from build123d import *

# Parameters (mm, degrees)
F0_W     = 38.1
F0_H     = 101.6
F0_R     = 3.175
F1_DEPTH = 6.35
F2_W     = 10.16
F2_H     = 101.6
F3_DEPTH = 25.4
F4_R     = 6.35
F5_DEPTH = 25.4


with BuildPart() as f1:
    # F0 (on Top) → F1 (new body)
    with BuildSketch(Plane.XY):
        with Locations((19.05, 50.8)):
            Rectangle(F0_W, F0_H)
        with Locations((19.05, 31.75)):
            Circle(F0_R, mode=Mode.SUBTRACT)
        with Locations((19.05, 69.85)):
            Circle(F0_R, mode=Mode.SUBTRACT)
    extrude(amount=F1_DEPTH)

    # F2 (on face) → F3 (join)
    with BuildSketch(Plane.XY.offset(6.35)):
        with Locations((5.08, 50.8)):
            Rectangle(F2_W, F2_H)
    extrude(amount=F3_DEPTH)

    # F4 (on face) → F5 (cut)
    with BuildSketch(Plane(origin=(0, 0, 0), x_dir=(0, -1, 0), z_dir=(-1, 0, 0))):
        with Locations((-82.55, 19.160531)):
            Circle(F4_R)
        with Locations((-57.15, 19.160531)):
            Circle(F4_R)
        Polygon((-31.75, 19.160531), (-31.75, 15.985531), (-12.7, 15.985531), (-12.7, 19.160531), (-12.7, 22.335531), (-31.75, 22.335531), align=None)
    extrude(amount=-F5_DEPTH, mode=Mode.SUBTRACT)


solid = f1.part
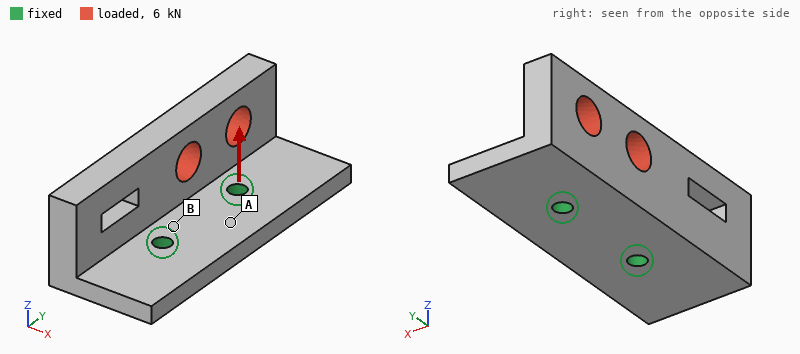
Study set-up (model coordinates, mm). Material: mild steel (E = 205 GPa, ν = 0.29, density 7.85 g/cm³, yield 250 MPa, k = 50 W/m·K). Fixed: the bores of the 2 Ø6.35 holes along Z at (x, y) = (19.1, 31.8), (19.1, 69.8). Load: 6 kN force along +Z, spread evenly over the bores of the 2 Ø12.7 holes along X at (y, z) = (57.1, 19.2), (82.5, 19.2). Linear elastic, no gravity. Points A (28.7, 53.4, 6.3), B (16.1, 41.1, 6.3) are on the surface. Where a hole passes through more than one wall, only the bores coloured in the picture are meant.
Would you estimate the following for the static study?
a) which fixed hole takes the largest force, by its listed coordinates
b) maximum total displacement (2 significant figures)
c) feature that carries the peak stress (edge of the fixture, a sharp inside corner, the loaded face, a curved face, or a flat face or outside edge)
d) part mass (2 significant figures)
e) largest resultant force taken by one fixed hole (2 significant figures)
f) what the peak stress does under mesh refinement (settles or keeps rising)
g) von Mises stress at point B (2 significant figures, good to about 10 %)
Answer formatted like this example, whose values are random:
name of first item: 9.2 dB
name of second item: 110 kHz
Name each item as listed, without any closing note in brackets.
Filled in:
which fixed hole takes the largest force, by its listed coordinates: (19.1, 69.8)
maximum total displacement: 92 µm
feature that carries the peak stress: edge of the fixture
part mass: 370 g
largest resultant force taken by one fixed hole: 5.5 kN
what the peak stress does under mesh refinement: keeps rising
von Mises stress at point B: 58 MPa
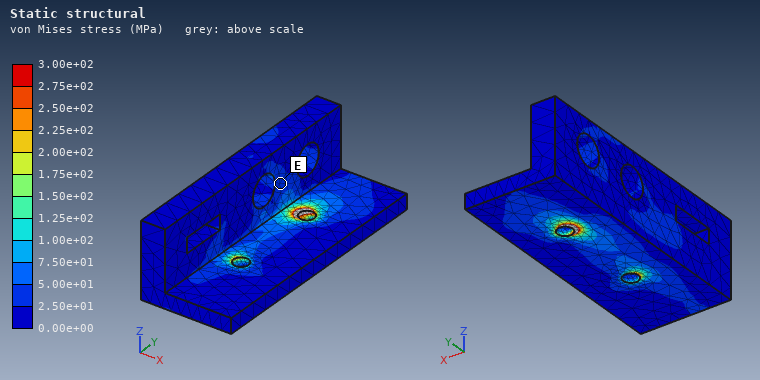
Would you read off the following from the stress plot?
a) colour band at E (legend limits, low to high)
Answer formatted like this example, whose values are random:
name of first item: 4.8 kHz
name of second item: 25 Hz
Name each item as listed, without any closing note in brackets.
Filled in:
colour band at E: 2.50e+01 to 5.00e+01 MPa
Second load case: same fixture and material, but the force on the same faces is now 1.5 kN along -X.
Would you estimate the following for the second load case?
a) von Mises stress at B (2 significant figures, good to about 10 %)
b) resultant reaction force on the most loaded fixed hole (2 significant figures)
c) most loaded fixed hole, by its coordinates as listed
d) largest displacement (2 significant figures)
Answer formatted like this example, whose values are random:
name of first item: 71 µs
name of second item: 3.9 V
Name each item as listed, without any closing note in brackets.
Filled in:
von Mises stress at B: 25 MPa
resultant reaction force on the most loaded fixed hole: 1.4 kN
most loaded fixed hole, by its coordinates as listed: (19.1, 69.8)
largest displacement: 38 µm
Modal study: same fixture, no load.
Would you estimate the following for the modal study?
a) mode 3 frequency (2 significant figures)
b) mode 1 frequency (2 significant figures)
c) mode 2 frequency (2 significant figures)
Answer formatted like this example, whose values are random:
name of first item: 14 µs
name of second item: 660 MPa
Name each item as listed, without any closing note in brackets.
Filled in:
mode 3 frequency: 5900 Hz
mode 1 frequency: 3000 Hz
mode 2 frequency: 4000 Hz
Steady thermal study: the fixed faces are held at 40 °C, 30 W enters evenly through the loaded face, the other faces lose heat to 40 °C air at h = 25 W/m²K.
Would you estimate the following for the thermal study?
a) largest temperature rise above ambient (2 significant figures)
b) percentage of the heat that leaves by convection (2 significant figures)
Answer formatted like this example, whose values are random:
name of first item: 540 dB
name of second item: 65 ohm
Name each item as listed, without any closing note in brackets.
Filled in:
largest temperature rise above ambient: 39 K
percentage of the heat that leaves by convection: 18 %
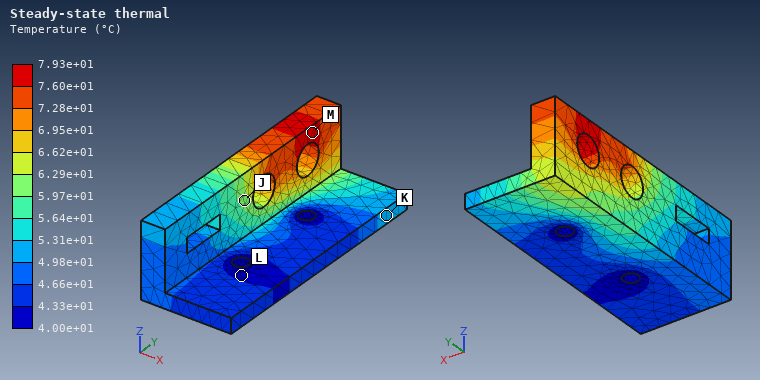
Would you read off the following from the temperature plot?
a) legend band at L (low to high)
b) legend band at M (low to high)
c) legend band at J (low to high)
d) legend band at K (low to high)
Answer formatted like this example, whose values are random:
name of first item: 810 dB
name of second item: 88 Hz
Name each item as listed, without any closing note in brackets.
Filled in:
legend band at L: 4.00e+01 to 4.33e+01 °C
legend band at M: 7.60e+01 to 7.93e+01 °C
legend band at J: 5.97e+01 to 6.29e+01 °C
legend band at K: 4.98e+01 to 5.31e+01 °C
